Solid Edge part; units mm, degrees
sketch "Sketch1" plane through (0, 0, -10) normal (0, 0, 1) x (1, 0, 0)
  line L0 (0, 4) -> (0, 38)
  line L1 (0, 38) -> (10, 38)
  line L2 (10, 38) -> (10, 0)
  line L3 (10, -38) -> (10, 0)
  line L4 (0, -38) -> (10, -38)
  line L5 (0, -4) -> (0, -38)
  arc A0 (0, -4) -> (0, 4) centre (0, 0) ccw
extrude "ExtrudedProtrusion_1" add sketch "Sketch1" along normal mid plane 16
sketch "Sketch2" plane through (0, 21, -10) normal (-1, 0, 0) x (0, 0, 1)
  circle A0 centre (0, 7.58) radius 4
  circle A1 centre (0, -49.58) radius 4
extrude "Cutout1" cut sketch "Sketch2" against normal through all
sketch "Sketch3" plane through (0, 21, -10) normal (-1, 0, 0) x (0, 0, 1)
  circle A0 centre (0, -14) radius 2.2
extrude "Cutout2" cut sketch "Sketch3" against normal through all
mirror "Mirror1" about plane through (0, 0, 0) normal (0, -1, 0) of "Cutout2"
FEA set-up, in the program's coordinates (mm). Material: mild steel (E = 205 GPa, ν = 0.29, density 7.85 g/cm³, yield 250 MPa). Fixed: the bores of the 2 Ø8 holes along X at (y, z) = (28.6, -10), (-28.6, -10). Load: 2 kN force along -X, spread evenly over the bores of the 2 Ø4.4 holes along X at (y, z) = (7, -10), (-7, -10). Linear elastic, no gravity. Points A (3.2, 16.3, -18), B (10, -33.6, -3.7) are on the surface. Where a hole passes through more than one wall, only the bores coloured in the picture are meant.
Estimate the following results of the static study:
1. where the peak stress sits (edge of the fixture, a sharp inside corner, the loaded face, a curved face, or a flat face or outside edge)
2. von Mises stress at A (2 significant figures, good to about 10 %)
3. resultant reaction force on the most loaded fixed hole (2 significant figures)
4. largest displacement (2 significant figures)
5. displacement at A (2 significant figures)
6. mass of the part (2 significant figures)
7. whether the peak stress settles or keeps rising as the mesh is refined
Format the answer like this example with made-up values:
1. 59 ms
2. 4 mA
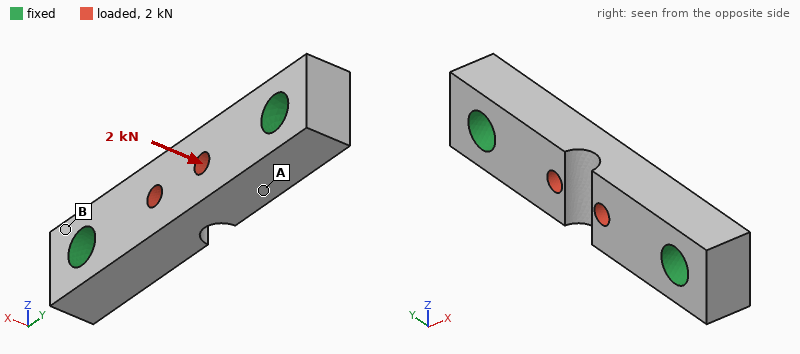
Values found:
1. edge of the fixture
2. 17 MPa
3. 1.1 kN
4. 8.7 µm
5. 2.8 µm
6. 82 g
7. keeps rising
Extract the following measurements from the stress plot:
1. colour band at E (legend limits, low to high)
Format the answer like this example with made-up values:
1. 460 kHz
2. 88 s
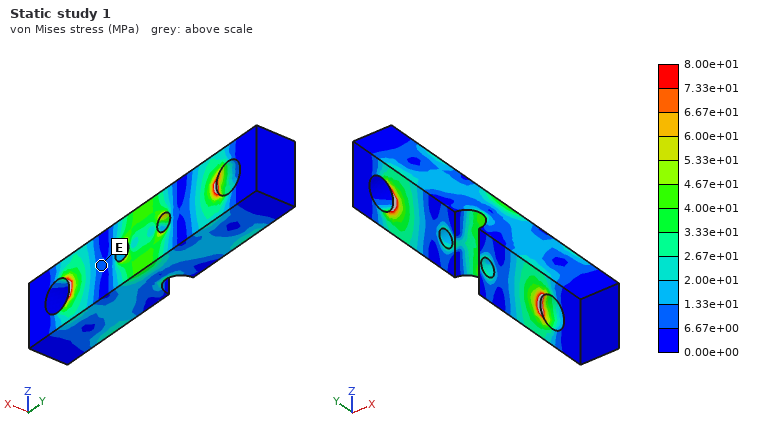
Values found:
1. 6.67e+00 to 1.33e+01 MPa
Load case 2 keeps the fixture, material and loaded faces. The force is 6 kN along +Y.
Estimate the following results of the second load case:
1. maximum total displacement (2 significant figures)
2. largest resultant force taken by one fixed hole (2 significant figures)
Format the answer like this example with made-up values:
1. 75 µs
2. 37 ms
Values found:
1. 3.7 µm
2. 3.0 kN
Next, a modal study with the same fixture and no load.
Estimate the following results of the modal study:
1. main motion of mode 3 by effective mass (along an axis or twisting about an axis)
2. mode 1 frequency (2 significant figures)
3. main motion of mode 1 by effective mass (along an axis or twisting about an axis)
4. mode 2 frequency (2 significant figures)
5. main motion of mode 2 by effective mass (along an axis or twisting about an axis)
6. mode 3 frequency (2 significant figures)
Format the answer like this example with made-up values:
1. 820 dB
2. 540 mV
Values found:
1. twisting about Y
2. 15 kHz
3. along X
4. 19 kHz
5. along Z
6. 27 kHz
